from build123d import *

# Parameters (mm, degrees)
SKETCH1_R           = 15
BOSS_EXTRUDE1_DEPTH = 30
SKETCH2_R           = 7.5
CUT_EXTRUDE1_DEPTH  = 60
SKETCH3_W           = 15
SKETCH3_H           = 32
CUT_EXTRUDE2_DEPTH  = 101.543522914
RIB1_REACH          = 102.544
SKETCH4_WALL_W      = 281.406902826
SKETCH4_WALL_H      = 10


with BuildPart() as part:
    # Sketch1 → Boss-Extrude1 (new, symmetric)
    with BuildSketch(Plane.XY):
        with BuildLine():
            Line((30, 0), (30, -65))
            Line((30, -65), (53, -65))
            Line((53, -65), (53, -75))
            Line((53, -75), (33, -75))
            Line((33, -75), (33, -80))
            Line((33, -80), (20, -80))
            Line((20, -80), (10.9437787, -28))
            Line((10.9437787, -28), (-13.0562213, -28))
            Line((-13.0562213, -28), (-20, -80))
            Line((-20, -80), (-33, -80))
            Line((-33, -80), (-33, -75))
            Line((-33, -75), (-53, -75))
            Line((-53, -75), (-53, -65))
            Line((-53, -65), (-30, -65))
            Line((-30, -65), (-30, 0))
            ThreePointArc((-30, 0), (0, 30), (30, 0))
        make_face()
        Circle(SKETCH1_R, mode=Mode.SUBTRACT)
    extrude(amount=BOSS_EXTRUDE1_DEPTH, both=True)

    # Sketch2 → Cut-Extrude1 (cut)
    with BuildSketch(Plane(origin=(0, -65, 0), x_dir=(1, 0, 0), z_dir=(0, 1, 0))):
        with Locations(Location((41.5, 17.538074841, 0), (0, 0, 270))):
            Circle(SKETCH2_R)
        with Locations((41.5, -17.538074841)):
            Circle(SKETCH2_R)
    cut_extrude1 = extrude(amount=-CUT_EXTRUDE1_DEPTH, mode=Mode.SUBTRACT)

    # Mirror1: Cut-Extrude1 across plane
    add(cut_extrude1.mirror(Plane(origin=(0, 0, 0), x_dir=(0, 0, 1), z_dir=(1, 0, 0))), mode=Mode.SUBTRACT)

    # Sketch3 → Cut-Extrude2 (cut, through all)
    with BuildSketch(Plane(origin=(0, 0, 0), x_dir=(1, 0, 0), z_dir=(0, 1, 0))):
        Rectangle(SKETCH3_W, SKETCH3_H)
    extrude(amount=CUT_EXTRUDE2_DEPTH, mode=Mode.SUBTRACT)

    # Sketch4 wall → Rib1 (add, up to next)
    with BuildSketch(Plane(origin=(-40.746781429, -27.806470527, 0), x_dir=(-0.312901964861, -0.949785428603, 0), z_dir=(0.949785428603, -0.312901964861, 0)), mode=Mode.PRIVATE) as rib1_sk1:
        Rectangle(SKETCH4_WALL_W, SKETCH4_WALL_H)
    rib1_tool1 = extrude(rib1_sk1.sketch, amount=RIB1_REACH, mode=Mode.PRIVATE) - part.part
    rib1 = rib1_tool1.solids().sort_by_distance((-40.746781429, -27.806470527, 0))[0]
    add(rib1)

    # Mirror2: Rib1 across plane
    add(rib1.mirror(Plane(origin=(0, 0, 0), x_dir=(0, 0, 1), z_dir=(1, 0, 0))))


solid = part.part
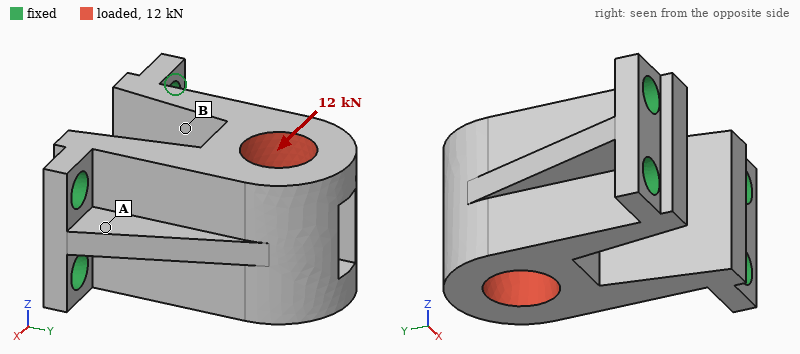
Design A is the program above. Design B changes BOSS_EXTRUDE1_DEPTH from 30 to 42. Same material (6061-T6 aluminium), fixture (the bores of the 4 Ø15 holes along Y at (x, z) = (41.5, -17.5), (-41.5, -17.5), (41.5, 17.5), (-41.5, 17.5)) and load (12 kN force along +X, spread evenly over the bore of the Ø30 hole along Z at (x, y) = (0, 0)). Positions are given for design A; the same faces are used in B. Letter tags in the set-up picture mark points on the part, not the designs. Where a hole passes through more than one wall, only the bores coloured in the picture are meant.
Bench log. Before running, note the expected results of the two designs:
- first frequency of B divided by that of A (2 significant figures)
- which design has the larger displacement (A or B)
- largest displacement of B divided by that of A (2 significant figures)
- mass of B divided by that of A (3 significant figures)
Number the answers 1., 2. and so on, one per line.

1. 0.95
2. A
3. 0.82
4. 1.40
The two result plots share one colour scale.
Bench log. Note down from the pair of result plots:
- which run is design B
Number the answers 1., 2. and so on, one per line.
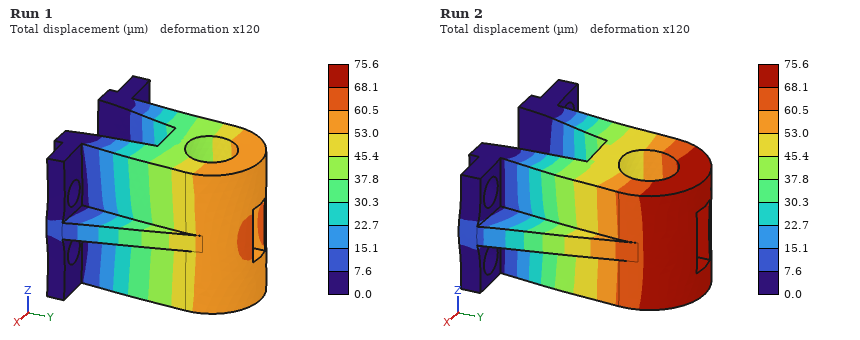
1. Run 1
